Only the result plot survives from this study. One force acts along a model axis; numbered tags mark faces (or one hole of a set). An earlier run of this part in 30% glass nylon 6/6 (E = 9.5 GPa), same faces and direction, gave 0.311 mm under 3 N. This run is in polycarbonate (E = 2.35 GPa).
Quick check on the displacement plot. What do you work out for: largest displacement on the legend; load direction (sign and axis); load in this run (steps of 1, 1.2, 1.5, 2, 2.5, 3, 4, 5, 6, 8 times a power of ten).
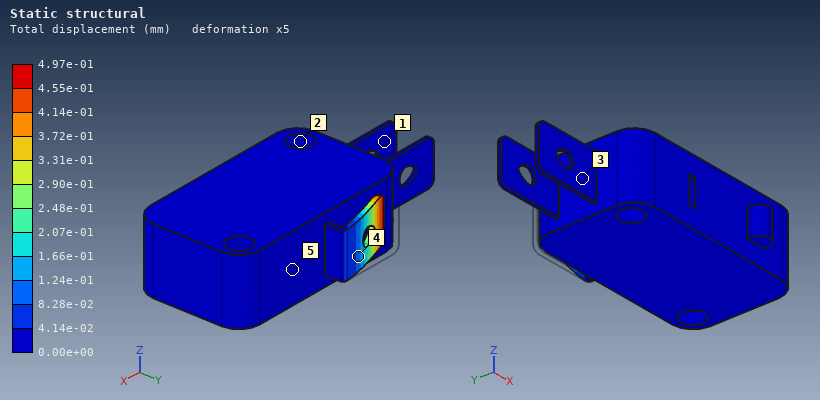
4.97e-01 mm
-Y
1.2 N
